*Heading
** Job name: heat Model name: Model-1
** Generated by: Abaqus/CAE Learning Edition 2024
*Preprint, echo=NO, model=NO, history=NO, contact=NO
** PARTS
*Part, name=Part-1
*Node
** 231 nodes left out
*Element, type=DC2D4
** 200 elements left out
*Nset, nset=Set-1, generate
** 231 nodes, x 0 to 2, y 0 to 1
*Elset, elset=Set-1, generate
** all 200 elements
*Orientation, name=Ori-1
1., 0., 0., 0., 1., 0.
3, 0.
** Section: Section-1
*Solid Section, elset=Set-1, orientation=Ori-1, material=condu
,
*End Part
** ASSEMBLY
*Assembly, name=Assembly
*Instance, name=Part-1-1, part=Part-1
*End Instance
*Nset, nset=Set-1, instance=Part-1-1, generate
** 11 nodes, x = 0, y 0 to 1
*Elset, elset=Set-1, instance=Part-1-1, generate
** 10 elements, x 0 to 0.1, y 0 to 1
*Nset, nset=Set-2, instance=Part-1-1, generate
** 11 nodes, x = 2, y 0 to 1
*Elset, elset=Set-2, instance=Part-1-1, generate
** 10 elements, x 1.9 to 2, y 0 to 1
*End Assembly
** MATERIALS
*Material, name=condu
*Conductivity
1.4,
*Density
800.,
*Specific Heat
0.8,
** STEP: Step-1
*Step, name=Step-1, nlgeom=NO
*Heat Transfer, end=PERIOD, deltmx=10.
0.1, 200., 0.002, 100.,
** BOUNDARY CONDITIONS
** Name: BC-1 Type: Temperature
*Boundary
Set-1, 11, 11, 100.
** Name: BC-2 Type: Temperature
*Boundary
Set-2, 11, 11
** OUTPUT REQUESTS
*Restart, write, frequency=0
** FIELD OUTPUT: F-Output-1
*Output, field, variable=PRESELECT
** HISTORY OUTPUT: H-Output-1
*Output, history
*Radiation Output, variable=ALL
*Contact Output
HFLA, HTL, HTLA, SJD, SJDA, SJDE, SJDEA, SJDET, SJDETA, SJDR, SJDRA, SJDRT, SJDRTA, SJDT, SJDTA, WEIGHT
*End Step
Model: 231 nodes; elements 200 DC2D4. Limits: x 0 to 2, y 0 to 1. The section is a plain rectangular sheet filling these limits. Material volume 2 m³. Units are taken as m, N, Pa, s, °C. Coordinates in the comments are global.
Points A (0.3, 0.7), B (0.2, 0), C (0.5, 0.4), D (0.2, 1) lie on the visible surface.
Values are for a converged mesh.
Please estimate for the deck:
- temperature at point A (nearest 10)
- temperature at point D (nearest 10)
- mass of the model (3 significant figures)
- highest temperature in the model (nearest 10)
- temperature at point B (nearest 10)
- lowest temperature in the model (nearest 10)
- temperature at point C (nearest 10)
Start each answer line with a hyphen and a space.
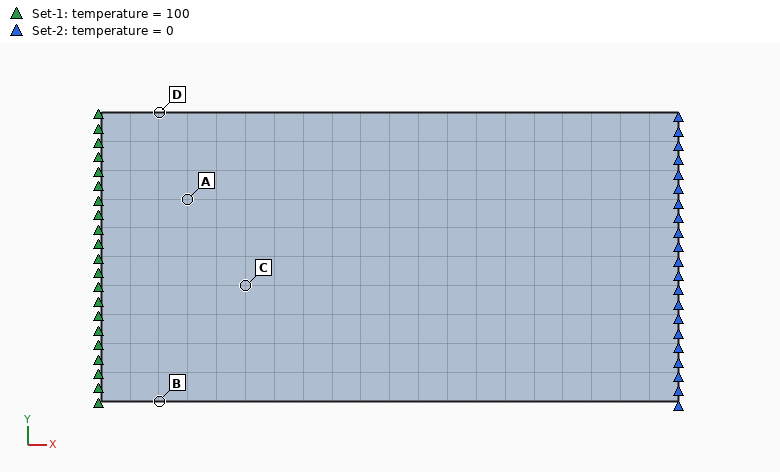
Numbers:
- 70 °C
- 80 °C
- 1600 kg
- 100 °C
- 80 °C
- 0 °C
- 60 °C
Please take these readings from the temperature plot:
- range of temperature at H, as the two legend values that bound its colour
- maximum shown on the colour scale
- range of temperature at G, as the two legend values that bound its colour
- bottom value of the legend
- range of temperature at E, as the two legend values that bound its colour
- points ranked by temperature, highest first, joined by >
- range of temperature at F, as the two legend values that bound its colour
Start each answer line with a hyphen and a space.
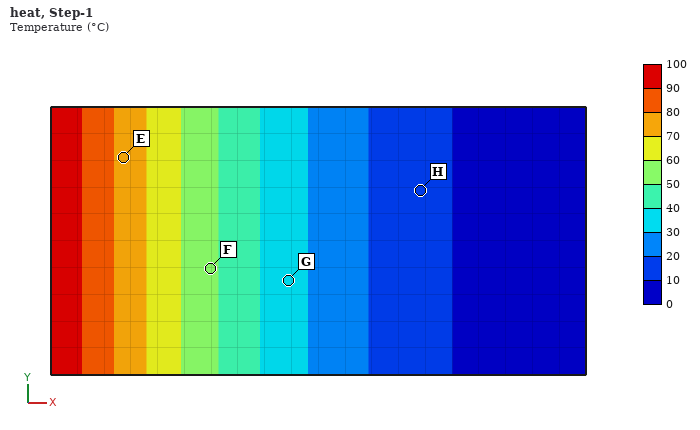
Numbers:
- 10 to 20 °C
- 100 °C
- 30 to 40 °C
- 0 °C
- 70 to 80 °C
- E > F > G > H
- 50 to 60 °C
